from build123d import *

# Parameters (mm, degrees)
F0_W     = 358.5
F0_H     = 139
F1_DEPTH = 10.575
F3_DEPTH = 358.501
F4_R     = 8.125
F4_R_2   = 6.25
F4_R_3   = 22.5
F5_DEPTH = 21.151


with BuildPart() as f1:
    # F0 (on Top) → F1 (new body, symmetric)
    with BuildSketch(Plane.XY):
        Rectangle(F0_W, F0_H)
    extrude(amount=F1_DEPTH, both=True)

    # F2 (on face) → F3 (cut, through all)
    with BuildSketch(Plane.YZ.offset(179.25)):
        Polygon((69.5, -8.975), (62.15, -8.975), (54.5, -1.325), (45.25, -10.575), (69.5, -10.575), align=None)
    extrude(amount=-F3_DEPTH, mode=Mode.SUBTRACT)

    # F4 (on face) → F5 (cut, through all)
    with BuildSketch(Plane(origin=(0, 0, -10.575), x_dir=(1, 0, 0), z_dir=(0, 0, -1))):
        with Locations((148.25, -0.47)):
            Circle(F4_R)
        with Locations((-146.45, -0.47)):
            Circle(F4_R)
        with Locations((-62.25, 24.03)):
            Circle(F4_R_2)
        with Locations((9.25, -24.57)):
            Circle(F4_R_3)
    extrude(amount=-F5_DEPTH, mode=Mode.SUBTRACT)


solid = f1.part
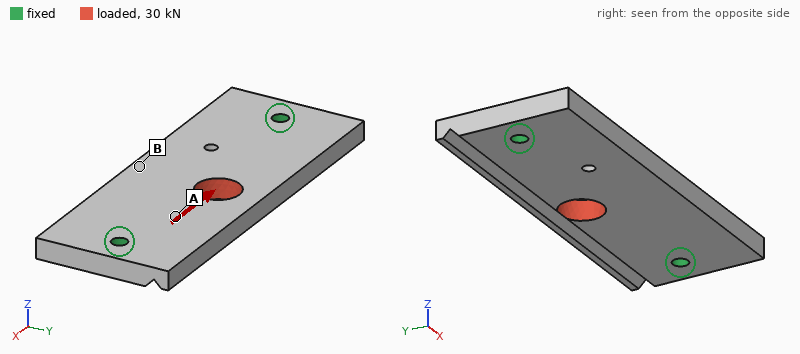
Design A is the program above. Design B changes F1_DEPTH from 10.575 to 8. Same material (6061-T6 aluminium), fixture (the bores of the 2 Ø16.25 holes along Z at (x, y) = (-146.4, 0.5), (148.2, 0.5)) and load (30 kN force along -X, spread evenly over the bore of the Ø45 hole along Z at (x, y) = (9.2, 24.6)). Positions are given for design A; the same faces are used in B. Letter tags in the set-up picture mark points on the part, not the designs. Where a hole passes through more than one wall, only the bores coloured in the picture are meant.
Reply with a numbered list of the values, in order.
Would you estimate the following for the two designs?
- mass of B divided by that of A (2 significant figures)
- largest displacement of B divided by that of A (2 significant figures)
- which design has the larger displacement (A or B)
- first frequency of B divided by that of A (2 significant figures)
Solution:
1. 0.77
2. 1.3
3. B
4. 0.79
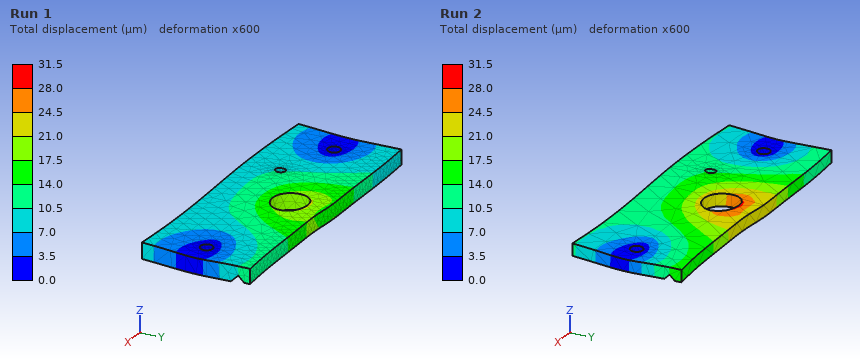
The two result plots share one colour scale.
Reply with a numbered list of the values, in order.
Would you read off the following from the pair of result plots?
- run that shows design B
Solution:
1. Run 2
